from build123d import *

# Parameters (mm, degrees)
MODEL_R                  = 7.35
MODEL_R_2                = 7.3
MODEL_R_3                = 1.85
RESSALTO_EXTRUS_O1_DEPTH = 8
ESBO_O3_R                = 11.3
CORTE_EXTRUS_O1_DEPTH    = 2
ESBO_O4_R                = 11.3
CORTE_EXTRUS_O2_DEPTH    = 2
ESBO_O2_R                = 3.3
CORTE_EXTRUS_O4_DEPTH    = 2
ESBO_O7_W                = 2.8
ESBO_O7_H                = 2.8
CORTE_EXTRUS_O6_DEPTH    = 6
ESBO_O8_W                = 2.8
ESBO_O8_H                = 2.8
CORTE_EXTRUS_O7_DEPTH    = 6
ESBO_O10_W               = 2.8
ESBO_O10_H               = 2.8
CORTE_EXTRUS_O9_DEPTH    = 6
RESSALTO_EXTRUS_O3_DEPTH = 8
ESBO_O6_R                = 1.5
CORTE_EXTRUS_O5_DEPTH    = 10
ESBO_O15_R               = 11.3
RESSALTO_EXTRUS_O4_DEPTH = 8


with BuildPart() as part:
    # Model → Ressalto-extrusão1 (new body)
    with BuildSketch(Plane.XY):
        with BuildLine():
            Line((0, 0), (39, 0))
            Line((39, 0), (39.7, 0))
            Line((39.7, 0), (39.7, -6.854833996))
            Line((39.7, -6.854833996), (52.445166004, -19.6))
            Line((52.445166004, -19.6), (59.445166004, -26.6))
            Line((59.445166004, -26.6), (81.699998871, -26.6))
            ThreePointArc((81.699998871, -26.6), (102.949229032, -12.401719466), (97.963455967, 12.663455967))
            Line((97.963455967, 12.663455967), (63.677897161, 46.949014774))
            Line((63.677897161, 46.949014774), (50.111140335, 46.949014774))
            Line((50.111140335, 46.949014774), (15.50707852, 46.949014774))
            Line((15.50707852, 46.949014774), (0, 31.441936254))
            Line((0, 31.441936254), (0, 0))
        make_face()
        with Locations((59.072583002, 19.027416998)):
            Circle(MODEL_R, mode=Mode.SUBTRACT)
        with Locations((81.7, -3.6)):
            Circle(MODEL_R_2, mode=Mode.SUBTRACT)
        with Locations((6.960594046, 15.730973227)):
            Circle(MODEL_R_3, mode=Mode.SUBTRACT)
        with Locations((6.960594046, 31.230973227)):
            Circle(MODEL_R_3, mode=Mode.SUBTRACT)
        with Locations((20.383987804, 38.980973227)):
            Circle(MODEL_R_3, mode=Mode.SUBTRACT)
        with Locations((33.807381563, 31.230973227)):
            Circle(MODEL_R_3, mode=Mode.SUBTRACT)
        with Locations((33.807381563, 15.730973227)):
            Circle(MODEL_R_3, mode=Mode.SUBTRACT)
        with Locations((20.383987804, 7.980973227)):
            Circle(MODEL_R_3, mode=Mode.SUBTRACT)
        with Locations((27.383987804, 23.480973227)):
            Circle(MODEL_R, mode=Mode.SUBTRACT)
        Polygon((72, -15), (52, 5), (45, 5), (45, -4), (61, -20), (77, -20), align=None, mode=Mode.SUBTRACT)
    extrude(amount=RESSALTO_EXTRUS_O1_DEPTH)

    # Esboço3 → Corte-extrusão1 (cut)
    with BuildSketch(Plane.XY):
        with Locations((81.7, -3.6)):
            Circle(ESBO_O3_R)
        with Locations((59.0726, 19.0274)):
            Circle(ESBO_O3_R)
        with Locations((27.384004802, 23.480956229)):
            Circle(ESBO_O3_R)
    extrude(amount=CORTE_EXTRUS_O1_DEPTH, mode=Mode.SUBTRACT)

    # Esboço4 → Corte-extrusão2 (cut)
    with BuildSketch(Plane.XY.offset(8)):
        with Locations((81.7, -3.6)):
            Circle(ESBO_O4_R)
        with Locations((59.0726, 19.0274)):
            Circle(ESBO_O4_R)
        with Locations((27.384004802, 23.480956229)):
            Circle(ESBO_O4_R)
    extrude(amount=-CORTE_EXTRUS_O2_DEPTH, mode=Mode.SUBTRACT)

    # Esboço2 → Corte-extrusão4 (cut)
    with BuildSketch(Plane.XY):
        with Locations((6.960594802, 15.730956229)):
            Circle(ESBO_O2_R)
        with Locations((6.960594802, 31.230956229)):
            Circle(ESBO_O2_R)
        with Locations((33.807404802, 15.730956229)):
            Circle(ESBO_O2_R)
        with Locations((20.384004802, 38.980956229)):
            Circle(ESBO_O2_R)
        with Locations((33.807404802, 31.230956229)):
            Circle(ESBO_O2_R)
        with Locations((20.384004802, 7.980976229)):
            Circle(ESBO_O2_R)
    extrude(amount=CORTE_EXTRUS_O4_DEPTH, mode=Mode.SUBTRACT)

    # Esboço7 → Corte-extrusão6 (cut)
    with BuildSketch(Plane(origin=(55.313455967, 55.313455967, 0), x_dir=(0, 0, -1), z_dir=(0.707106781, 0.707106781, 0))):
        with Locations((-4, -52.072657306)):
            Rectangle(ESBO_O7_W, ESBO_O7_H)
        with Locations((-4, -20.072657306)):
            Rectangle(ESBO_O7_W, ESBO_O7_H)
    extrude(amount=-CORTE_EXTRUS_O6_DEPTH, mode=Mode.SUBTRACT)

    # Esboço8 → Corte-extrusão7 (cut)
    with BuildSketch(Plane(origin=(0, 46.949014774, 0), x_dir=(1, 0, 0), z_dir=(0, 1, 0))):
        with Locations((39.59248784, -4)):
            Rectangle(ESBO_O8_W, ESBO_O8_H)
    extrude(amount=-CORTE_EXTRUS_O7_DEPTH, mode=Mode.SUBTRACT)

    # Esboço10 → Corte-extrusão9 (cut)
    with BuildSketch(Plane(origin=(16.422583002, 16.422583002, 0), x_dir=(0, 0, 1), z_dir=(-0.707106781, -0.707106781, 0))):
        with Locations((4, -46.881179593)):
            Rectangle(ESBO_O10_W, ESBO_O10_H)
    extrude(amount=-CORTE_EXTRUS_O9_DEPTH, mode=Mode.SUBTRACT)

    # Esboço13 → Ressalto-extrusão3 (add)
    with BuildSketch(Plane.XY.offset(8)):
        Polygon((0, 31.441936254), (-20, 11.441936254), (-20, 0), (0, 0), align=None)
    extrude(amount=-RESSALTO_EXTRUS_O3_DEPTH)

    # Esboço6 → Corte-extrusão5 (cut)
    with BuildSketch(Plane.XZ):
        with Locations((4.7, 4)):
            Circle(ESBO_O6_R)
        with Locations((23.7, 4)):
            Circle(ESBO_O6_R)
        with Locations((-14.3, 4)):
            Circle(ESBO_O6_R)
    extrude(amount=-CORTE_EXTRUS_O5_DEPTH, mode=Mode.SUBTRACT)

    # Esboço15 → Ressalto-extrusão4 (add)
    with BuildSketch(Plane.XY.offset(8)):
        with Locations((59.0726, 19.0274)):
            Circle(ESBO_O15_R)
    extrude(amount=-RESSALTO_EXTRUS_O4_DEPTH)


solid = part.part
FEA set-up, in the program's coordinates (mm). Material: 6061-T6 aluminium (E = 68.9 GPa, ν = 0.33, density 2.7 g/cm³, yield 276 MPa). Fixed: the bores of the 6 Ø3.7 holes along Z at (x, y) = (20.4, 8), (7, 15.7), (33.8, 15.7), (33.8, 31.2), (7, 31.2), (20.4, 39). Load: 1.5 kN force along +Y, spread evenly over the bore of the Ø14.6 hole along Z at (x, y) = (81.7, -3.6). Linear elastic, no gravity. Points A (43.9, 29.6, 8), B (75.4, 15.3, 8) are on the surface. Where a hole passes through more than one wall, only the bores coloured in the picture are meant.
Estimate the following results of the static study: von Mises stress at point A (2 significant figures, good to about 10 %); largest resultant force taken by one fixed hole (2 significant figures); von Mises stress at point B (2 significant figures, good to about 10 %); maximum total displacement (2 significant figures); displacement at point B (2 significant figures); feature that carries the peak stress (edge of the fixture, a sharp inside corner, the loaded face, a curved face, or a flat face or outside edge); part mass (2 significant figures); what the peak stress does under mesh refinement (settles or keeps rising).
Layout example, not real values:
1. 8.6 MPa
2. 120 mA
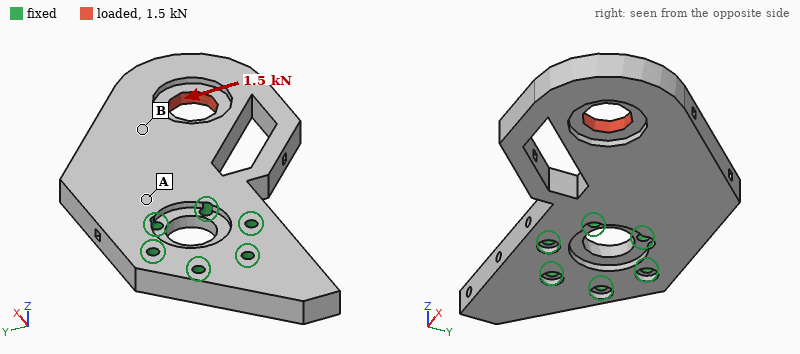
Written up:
1. 17 MPa
2. 1.7 kN
3. 7.7 MPa
4. 61 µm
5. 29 µm
6. edge of the fixture
7. 100 g
8. keeps rising
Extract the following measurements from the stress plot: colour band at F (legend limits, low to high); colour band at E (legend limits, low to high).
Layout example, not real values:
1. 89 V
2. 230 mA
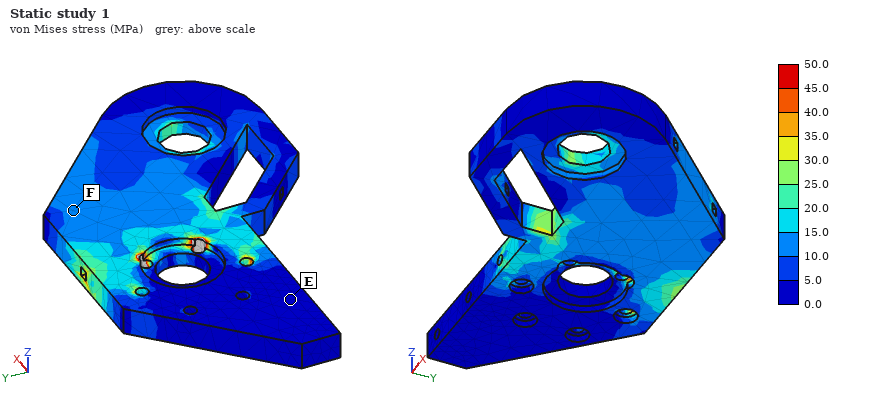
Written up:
1. 10.0 to 15.0 MPa
2. 0.0 to 5.0 MPa
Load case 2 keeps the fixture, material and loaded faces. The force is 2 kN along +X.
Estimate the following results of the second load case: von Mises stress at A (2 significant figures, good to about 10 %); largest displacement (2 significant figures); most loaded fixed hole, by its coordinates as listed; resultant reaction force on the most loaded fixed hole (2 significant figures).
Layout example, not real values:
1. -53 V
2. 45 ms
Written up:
1. 4.8 MPa
2. 60 µm
3. (33.8, 15.7)
4. 1.8 kN
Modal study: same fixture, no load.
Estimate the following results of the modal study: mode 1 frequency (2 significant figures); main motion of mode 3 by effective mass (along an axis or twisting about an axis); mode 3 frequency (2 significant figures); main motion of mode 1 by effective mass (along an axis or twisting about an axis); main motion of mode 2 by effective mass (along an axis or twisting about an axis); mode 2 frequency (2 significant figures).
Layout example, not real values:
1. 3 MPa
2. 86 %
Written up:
1. 1100 Hz
2. along Y
3. 4300 Hz
4. along Z
5. twisting about X
6. 3000 Hz
